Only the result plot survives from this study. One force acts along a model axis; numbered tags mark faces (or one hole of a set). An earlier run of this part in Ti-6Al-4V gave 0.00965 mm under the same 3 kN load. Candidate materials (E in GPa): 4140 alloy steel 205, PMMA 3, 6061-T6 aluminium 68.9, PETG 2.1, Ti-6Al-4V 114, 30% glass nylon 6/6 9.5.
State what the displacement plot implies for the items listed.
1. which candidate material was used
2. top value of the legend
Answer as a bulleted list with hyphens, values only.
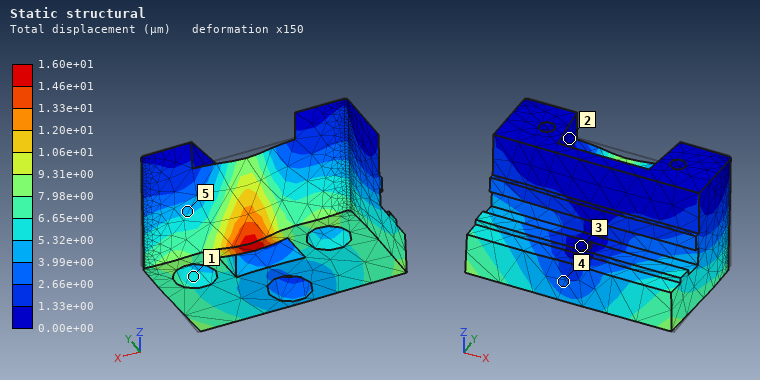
- 6061-T6 aluminium
- 1.60e+01 µm
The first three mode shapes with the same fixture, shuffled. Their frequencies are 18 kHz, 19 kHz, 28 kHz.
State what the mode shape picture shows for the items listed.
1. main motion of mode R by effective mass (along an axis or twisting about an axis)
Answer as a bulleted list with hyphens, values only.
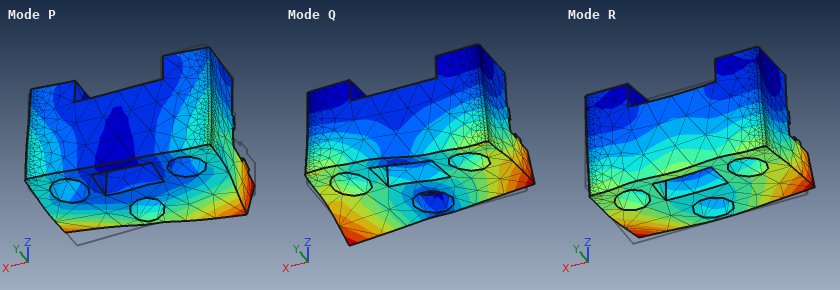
- along Y
